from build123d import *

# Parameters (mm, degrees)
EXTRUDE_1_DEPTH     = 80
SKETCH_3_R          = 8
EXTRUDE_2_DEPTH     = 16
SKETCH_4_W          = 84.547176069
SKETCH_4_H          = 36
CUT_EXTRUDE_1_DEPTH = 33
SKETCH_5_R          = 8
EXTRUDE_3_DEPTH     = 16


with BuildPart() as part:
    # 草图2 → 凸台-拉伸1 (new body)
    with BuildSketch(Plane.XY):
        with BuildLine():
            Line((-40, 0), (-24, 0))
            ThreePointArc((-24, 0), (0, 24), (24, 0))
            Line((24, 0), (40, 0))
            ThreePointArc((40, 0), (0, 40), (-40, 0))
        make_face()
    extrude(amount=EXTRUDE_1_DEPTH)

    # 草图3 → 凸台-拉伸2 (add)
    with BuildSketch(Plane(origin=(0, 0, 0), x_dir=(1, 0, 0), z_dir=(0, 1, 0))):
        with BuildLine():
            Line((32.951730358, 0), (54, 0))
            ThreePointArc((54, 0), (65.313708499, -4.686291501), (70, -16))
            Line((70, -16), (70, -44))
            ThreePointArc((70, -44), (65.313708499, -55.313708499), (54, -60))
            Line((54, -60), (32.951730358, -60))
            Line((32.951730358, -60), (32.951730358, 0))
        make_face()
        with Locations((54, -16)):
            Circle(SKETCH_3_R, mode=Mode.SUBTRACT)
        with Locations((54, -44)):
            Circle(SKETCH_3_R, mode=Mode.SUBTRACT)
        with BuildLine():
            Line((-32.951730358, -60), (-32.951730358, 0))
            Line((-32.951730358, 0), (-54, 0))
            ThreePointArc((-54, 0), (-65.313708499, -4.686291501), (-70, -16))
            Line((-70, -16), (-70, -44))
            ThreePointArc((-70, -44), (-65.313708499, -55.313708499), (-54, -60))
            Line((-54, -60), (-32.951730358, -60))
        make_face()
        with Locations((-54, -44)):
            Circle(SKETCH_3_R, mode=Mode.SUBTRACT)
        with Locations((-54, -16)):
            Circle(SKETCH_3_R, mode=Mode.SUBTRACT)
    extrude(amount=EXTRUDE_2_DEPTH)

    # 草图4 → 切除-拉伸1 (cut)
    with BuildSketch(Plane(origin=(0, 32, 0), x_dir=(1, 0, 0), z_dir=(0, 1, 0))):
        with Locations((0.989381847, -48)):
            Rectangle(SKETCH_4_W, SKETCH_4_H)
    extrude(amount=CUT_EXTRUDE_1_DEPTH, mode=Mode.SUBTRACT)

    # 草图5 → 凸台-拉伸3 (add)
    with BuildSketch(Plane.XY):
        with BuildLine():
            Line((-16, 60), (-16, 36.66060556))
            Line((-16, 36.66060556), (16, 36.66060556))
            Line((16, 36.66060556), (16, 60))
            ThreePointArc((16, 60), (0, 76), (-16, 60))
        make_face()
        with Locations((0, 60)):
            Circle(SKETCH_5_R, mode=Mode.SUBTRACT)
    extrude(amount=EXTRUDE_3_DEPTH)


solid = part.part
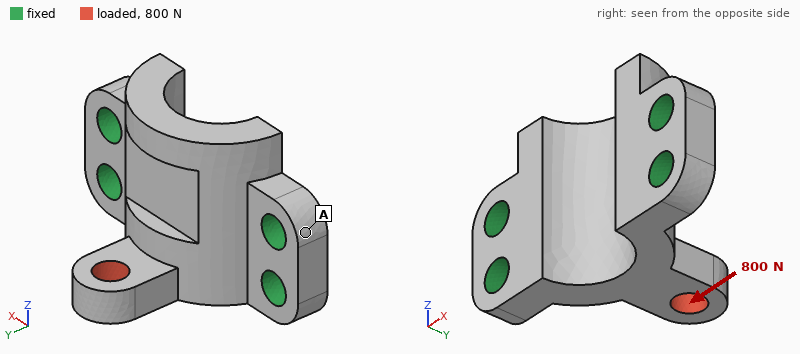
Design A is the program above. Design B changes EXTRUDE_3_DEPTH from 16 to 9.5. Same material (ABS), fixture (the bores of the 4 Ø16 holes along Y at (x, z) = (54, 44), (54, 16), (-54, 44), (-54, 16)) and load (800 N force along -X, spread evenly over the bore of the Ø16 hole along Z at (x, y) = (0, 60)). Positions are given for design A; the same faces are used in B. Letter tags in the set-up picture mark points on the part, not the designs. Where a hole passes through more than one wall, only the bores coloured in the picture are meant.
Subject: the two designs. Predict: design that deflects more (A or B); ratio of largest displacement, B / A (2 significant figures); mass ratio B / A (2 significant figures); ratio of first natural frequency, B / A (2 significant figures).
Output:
B
1.5
0.97
0.97
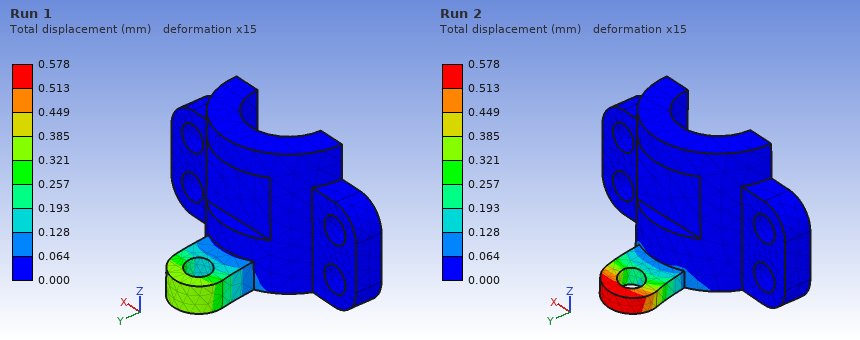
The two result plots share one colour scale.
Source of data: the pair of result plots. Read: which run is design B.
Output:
Run 2
